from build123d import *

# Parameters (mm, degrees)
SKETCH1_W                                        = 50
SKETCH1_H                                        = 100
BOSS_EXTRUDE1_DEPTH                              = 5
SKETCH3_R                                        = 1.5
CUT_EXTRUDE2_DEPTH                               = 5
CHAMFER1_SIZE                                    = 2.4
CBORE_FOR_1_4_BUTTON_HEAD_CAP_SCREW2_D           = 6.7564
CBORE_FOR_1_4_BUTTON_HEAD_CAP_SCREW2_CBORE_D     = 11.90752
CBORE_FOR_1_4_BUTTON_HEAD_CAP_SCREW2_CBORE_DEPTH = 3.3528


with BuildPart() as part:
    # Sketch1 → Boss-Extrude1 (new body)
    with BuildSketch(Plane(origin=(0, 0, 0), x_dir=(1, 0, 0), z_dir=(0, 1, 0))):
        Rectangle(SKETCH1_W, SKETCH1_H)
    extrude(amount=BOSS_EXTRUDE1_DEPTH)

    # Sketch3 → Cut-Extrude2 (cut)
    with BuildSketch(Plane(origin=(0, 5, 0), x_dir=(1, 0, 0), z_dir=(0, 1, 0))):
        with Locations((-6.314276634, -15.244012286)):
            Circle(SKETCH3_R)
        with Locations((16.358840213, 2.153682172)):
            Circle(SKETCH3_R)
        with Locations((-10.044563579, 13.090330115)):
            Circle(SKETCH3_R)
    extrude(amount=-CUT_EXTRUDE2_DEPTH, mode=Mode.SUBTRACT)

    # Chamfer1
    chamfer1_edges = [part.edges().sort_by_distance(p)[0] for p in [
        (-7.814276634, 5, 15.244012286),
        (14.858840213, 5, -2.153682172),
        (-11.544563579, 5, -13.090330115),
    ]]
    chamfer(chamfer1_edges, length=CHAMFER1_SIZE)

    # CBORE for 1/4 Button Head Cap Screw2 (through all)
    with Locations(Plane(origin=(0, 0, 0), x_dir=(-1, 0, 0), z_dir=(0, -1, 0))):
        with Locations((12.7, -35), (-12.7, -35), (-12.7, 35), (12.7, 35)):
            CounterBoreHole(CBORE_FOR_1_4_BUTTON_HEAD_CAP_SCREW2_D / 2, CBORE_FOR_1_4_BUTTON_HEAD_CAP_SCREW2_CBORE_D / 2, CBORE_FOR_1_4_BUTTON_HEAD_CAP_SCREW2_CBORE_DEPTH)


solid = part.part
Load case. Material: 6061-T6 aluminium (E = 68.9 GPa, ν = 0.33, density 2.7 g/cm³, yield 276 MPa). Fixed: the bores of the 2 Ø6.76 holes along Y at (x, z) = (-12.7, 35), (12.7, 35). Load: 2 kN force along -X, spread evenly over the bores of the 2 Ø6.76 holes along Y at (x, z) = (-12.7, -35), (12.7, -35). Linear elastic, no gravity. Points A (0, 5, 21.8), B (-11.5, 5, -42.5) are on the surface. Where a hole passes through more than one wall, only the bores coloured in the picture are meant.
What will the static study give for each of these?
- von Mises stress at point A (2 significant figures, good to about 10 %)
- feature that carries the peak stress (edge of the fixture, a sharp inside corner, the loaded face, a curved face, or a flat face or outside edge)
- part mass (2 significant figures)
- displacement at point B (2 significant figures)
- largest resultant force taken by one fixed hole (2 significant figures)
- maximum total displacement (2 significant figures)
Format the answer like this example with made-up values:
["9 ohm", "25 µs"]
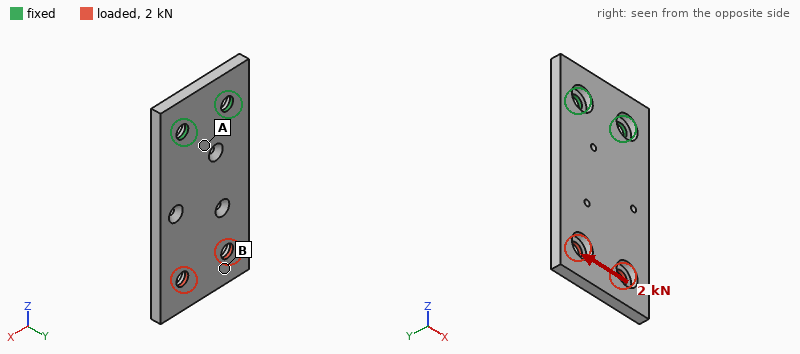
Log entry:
["64 MPa", "edge of the fixture", "62 g", "0.22 mm", "4.9 kN", "0.29 mm"]
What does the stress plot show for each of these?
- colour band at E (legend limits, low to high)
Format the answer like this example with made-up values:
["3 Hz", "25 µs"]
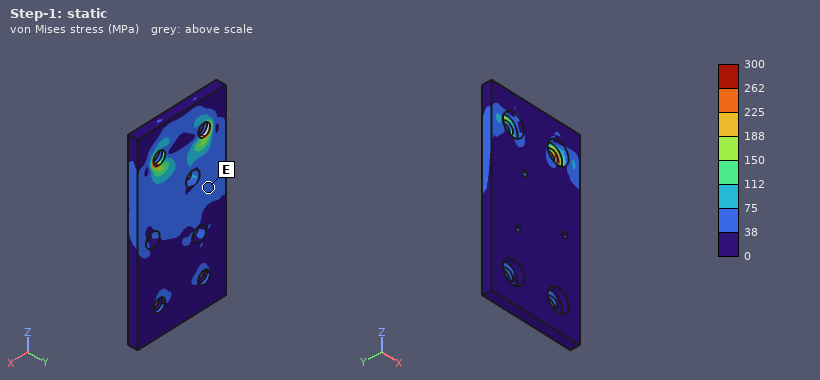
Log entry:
["38 to 75 MPa"]
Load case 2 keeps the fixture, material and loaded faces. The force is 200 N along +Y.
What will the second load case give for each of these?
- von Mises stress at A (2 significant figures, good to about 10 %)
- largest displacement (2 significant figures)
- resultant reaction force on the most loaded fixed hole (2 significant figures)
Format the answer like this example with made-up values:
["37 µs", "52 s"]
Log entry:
["55 MPa", "1.3 mm", "240 N"]
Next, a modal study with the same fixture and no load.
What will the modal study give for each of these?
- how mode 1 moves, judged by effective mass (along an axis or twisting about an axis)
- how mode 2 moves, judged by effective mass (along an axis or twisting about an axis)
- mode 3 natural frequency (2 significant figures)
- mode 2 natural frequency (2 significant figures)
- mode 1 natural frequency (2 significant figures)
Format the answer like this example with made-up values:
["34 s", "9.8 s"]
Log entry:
["along Y", "twisting about Z", "2900 Hz", "1900 Hz", "470 Hz"]
